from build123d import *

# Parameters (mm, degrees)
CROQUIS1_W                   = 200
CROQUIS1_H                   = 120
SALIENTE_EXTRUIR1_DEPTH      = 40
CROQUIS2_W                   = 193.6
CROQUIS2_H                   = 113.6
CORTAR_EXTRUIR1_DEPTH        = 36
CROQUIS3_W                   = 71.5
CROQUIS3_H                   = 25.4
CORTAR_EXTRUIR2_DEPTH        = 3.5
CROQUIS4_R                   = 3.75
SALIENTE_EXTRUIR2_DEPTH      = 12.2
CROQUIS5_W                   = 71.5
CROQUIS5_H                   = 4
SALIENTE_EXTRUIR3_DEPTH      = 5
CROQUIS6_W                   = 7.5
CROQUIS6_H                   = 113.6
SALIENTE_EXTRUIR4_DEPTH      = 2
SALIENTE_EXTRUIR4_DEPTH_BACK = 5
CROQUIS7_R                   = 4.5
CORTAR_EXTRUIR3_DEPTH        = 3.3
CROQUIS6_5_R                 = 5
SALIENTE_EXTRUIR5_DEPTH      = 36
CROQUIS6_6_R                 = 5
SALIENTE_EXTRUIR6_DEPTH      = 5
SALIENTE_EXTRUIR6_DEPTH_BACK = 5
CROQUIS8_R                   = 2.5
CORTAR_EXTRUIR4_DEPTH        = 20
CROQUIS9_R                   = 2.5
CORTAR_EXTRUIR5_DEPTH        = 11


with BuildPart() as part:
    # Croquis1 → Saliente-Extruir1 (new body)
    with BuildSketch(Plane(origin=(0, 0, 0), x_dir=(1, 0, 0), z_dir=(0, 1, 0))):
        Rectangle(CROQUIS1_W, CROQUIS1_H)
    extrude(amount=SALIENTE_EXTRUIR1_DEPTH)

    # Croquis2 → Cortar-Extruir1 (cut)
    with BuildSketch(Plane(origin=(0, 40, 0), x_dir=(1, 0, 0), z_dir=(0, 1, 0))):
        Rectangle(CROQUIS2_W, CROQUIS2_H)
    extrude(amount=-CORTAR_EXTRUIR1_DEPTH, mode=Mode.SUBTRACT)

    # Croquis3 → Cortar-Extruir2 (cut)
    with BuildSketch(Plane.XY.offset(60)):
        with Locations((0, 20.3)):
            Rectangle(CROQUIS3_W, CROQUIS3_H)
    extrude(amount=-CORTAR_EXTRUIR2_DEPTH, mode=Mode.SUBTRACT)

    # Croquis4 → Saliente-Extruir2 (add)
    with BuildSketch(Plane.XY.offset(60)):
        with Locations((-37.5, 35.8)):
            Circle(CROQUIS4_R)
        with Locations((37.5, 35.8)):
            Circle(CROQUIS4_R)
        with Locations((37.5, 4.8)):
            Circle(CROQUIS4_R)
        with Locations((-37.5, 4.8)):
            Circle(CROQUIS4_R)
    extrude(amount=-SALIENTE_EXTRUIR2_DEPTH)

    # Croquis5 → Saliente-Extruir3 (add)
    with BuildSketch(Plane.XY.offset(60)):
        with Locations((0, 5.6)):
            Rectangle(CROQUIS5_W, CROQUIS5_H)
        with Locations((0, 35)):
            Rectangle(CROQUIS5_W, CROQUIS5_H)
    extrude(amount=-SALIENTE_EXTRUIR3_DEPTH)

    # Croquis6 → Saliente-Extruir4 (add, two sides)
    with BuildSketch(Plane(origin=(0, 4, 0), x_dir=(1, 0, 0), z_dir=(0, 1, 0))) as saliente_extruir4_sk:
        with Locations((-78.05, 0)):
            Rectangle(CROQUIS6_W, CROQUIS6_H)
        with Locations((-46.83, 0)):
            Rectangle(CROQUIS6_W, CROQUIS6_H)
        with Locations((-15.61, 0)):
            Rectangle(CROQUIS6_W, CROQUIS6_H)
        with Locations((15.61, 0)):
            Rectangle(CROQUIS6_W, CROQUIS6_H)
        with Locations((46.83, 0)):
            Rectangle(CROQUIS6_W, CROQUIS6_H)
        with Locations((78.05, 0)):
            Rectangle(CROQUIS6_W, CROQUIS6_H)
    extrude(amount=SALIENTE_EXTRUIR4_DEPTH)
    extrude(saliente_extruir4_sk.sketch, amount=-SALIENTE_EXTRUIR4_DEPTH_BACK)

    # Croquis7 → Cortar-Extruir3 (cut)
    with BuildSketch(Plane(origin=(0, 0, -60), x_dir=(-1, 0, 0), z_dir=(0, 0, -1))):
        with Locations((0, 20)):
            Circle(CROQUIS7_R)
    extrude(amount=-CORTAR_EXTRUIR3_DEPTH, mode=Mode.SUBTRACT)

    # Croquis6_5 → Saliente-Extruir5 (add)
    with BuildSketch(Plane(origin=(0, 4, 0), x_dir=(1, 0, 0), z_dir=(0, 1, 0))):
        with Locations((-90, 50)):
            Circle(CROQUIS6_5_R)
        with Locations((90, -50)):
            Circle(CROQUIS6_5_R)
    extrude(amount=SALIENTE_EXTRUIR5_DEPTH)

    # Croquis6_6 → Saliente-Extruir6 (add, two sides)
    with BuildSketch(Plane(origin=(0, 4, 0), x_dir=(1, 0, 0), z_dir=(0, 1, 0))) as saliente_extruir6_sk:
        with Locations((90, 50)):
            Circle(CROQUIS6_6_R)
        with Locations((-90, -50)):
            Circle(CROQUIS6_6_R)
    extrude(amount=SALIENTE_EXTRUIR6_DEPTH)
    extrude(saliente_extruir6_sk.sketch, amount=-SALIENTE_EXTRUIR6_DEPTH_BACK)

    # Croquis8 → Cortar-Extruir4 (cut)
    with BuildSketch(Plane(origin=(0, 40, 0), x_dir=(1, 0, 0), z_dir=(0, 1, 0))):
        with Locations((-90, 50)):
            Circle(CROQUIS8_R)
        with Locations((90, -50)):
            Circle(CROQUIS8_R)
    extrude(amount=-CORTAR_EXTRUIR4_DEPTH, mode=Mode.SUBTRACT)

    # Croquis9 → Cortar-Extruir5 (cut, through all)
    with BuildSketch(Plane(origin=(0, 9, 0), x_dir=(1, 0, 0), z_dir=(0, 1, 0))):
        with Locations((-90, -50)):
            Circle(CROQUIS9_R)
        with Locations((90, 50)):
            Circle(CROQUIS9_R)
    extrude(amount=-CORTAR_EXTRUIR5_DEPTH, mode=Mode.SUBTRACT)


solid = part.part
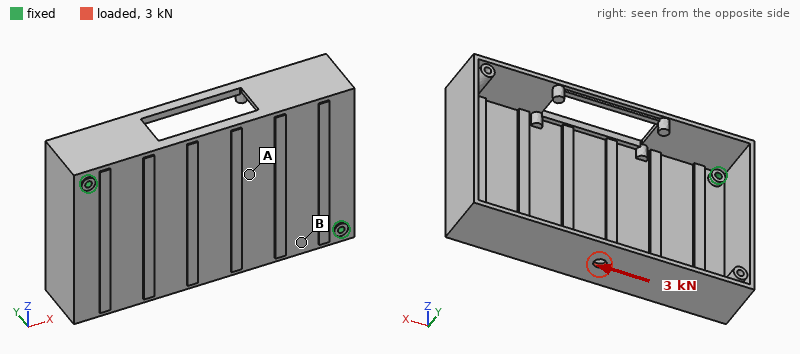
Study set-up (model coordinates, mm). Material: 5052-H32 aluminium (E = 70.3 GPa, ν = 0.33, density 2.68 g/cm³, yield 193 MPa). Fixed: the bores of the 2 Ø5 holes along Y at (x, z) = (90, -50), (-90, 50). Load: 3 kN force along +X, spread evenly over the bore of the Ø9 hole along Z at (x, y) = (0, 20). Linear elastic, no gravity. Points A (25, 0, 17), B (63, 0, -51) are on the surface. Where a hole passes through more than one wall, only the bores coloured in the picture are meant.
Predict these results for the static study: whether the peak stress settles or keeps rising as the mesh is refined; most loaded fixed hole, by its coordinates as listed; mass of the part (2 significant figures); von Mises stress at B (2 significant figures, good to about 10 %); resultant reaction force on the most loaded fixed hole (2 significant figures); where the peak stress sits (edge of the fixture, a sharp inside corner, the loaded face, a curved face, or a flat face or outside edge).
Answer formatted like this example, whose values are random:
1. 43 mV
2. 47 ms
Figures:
1. keeps rising
2. (90, -50)
3. 500 g
4. 13 MPa
5. 2.3 kN
6. edge of the fixture
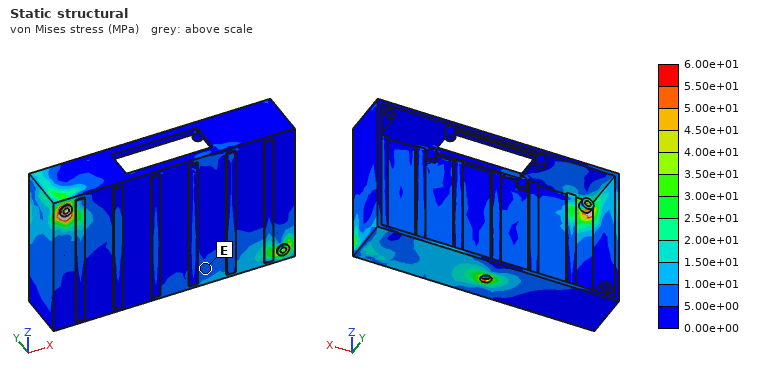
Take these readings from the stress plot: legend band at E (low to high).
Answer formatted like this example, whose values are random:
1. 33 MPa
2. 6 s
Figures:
1. 5.00e+00 to 1.00e+01 MPa
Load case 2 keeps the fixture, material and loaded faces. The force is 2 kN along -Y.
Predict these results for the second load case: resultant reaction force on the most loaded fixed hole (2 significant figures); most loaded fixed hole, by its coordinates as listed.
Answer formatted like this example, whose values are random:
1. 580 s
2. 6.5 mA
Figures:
1. 1.3 kN
2. (90, -50)
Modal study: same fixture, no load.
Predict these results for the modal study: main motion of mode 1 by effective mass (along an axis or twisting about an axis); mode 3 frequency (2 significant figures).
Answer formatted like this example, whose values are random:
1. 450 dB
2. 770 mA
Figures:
1. along Y
2. 1200 Hz
